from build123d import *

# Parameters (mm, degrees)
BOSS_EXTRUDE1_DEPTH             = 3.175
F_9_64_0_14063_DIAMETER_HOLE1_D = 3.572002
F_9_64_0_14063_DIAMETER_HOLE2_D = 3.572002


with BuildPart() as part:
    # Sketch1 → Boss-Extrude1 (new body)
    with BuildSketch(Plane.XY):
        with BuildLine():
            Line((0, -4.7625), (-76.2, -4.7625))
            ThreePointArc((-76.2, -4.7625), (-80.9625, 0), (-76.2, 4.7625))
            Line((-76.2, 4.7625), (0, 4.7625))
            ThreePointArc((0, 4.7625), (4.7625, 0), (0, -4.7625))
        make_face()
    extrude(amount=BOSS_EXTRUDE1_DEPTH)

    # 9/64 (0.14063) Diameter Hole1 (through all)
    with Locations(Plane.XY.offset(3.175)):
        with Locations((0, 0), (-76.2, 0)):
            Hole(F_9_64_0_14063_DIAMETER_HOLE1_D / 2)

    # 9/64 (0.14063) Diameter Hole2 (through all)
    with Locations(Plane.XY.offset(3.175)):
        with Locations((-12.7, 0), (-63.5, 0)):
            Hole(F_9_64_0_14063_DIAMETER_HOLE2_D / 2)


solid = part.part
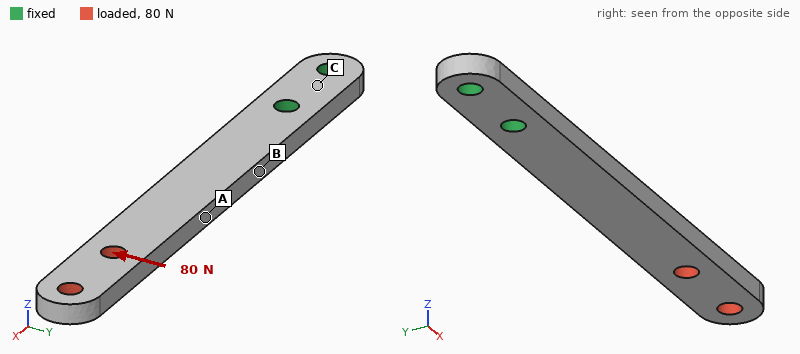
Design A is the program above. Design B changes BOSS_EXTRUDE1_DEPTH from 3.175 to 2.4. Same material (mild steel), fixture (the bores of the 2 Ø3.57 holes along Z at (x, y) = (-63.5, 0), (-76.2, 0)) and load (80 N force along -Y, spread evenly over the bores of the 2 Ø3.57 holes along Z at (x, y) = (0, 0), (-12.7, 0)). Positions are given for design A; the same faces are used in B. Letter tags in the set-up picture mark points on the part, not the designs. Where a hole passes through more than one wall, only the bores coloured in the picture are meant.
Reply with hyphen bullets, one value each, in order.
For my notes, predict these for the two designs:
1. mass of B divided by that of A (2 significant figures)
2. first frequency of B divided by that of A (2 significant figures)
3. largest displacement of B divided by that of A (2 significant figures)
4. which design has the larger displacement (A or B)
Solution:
- 0.76
- 0.76
- 1.3
- B
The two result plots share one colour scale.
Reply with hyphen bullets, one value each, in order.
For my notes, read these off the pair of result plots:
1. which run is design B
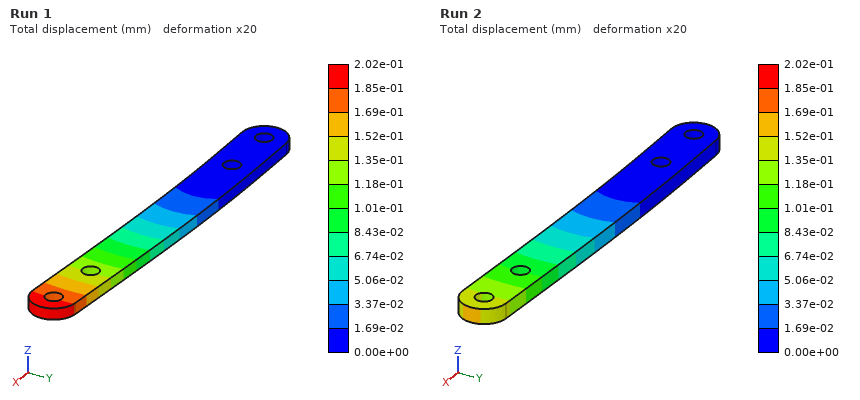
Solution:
- Run 1
